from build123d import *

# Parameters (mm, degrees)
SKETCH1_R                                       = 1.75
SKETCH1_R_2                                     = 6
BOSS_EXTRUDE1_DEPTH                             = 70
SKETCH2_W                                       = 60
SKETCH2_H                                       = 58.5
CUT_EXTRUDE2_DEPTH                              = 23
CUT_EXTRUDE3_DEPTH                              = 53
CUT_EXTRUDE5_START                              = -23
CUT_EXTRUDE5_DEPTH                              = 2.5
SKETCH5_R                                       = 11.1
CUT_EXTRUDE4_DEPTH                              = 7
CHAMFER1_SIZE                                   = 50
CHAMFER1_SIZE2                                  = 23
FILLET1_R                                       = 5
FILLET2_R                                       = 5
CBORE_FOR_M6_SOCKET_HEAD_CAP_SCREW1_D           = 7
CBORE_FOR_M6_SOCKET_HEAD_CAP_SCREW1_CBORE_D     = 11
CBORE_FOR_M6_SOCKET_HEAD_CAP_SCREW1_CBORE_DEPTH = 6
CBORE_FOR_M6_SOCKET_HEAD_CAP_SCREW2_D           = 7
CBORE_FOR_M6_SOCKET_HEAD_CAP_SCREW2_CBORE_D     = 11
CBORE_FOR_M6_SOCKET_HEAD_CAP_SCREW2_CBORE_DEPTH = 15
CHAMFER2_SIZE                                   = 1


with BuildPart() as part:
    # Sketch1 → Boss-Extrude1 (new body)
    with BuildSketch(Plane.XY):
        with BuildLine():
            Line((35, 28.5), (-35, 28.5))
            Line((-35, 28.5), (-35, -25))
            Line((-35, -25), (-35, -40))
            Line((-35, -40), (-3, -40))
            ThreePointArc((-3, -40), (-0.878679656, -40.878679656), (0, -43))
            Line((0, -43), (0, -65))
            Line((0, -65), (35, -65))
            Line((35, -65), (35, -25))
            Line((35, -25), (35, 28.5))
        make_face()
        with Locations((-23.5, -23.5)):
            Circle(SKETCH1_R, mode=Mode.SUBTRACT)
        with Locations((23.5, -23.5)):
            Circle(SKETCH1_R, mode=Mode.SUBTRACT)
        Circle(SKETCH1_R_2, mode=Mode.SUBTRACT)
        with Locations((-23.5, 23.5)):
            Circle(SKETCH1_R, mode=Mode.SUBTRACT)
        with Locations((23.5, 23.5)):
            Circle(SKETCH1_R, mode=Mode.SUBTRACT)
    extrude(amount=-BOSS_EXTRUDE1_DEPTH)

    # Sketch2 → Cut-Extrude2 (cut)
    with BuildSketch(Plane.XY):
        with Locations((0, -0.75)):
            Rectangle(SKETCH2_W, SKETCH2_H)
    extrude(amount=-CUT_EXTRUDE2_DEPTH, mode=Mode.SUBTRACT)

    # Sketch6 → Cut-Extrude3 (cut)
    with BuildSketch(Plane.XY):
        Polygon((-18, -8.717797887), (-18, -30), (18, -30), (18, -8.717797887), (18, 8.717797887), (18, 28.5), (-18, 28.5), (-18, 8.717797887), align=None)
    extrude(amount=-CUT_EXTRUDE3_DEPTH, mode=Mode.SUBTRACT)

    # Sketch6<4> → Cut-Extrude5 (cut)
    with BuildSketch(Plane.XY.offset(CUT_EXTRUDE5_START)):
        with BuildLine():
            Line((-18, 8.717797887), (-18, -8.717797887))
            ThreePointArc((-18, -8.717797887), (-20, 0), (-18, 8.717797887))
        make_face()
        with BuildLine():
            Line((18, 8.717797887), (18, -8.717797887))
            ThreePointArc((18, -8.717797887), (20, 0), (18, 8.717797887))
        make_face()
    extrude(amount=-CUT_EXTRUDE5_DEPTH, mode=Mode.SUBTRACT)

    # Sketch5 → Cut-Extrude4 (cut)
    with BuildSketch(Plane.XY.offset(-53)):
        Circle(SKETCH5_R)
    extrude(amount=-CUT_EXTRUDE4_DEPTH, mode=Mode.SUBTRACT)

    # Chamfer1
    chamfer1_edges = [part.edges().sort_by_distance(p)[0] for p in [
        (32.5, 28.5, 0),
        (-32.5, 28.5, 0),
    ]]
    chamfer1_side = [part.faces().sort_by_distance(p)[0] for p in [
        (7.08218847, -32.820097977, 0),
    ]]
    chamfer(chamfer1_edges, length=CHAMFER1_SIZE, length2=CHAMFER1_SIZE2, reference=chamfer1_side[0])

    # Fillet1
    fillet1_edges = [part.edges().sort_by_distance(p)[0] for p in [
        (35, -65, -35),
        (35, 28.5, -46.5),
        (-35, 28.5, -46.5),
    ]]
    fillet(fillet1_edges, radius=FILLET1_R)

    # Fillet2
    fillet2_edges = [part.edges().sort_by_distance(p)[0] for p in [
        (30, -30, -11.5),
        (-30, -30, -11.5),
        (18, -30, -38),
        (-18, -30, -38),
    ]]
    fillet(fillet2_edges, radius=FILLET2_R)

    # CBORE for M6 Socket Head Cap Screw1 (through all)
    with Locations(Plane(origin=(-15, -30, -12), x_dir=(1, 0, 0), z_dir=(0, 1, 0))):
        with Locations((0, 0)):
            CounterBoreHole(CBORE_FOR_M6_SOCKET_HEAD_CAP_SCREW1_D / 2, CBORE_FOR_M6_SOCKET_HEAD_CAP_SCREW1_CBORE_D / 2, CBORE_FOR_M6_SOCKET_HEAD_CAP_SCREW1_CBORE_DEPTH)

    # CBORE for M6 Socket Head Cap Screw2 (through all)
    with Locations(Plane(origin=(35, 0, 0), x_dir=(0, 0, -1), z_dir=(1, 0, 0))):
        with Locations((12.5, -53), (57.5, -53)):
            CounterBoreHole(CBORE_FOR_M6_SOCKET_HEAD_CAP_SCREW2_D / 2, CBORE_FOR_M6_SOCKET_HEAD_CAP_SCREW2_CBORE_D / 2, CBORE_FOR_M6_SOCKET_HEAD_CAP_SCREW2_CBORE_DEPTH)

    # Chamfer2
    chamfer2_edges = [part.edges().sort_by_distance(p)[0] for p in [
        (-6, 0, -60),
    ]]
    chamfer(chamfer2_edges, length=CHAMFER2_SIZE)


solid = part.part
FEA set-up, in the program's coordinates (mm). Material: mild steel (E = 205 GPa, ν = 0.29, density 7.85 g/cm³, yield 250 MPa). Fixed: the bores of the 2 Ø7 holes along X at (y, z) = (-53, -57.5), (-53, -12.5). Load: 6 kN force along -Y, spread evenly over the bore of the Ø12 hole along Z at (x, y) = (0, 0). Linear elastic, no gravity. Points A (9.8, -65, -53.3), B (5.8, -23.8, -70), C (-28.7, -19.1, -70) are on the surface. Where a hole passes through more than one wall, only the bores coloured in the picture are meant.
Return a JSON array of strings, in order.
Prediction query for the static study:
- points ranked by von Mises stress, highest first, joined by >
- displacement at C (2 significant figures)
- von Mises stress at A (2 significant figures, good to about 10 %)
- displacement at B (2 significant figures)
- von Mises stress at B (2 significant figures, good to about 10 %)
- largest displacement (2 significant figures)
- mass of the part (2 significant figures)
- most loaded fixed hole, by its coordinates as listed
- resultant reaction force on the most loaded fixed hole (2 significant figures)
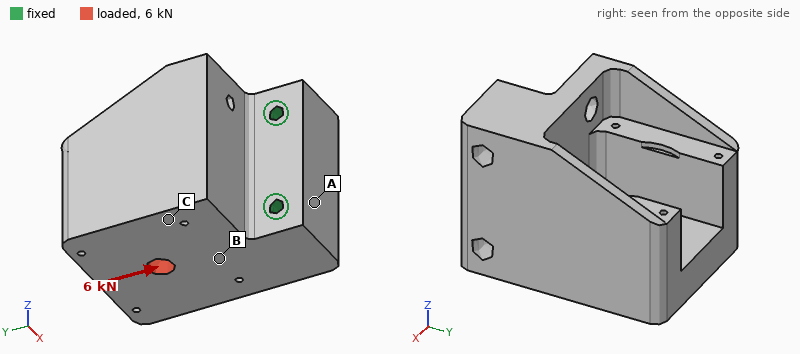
["B > A > C", "11 µm", "6.1 MPa", "4.4 µm", "16 MPa", "16 µm", "1.9 kg", "(-53, -57.5)", "6.9 kN"]
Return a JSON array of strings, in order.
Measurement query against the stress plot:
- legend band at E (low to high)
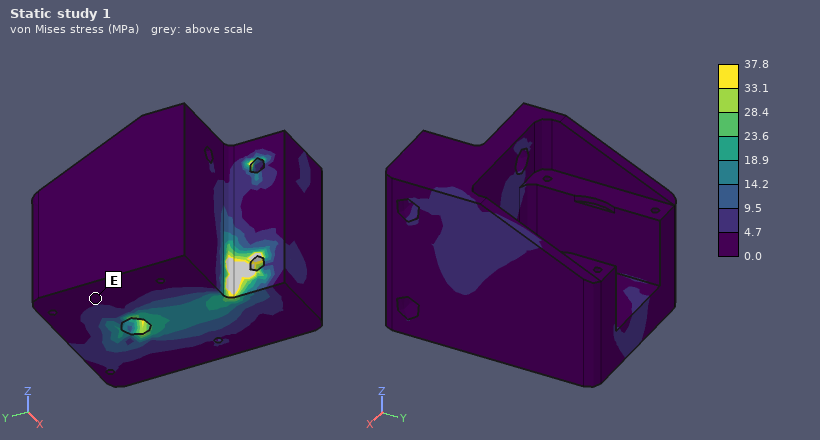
["0.0 to 4.7 MPa"]
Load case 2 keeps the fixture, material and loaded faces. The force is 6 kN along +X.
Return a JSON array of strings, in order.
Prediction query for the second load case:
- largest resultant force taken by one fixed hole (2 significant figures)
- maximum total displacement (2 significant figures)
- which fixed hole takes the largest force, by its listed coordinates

["6.3 kN", "54 µm", "(-53, -57.5)"]
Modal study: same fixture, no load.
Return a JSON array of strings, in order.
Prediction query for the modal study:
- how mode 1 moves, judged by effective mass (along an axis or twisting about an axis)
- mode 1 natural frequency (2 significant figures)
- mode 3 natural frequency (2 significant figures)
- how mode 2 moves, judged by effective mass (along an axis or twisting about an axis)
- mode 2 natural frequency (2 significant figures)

["along X", "1800 Hz", "5900 Hz", "along Z", "3300 Hz"]
